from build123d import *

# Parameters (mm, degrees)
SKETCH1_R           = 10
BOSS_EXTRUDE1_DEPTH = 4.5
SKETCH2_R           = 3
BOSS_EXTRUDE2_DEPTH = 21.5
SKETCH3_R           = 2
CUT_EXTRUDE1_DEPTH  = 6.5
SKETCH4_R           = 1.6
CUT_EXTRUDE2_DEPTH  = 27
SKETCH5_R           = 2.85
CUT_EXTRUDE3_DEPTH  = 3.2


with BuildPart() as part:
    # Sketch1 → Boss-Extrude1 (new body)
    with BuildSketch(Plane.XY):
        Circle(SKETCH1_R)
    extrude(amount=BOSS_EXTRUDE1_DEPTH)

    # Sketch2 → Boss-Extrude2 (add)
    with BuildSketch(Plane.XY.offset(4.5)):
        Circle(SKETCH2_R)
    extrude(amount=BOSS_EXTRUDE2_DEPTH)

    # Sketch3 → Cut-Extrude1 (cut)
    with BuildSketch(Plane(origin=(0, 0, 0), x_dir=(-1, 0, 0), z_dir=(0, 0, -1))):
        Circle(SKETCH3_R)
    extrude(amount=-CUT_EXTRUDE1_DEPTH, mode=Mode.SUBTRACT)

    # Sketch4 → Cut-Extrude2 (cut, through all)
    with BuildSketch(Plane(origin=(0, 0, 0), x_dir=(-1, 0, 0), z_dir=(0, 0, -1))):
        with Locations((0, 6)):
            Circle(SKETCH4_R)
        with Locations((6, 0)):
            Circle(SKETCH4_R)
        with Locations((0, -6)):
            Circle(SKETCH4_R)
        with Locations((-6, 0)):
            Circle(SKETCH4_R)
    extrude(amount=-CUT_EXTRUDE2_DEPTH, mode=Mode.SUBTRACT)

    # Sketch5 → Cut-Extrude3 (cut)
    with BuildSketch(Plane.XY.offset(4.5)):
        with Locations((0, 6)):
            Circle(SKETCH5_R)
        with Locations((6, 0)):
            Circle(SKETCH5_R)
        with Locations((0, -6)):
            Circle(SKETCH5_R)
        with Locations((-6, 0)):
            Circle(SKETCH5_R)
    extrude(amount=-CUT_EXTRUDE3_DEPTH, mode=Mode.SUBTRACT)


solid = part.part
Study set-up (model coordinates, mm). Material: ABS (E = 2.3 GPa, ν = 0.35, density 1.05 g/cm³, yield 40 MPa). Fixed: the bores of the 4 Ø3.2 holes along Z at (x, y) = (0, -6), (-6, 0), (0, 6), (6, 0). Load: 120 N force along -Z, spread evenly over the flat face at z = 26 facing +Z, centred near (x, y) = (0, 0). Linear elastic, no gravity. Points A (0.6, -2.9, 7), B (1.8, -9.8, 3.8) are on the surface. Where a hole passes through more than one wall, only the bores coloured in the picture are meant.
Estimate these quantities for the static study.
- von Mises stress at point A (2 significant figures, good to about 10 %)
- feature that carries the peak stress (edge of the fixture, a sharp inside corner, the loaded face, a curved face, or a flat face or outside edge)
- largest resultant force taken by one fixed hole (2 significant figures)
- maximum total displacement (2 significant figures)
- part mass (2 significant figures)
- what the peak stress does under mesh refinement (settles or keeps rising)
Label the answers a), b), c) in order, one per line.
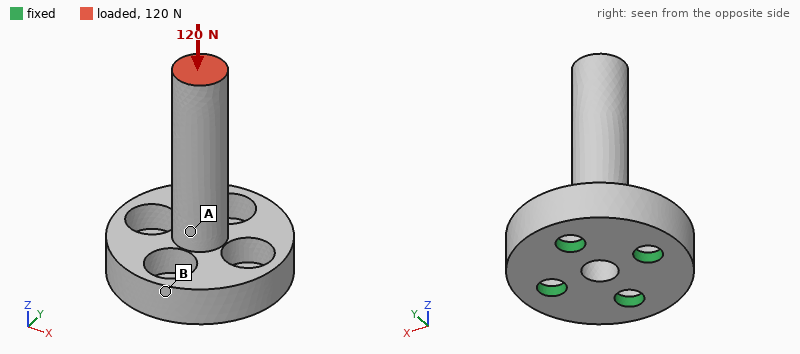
a) 6.2 MPa
b) edge of the fixture
c) 34 N
d) 61 µm
e) 1.7 g
f) keeps rising
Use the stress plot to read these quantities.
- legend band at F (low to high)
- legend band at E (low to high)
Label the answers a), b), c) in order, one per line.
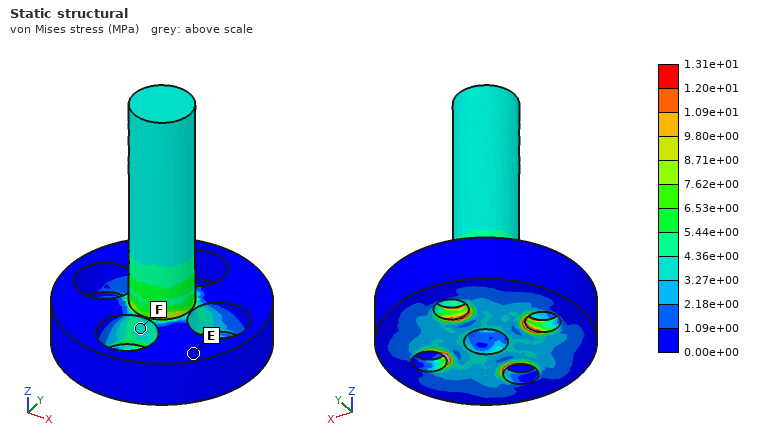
a) 3.27e+00 to 4.36e+00 MPa
b) 0.00e+00 to 1.09e+00 MPa
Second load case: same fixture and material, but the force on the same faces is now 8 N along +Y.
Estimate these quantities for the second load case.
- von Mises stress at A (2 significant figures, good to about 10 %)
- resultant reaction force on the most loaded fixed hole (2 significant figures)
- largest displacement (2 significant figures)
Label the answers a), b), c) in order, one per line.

a) 7.7 MPa
b) 17 N
c) 0.29 mm
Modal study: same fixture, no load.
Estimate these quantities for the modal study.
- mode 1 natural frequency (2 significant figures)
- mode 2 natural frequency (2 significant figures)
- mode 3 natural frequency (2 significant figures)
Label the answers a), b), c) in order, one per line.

a) 2000 Hz
b) 2000 Hz
c) 9500 Hz
